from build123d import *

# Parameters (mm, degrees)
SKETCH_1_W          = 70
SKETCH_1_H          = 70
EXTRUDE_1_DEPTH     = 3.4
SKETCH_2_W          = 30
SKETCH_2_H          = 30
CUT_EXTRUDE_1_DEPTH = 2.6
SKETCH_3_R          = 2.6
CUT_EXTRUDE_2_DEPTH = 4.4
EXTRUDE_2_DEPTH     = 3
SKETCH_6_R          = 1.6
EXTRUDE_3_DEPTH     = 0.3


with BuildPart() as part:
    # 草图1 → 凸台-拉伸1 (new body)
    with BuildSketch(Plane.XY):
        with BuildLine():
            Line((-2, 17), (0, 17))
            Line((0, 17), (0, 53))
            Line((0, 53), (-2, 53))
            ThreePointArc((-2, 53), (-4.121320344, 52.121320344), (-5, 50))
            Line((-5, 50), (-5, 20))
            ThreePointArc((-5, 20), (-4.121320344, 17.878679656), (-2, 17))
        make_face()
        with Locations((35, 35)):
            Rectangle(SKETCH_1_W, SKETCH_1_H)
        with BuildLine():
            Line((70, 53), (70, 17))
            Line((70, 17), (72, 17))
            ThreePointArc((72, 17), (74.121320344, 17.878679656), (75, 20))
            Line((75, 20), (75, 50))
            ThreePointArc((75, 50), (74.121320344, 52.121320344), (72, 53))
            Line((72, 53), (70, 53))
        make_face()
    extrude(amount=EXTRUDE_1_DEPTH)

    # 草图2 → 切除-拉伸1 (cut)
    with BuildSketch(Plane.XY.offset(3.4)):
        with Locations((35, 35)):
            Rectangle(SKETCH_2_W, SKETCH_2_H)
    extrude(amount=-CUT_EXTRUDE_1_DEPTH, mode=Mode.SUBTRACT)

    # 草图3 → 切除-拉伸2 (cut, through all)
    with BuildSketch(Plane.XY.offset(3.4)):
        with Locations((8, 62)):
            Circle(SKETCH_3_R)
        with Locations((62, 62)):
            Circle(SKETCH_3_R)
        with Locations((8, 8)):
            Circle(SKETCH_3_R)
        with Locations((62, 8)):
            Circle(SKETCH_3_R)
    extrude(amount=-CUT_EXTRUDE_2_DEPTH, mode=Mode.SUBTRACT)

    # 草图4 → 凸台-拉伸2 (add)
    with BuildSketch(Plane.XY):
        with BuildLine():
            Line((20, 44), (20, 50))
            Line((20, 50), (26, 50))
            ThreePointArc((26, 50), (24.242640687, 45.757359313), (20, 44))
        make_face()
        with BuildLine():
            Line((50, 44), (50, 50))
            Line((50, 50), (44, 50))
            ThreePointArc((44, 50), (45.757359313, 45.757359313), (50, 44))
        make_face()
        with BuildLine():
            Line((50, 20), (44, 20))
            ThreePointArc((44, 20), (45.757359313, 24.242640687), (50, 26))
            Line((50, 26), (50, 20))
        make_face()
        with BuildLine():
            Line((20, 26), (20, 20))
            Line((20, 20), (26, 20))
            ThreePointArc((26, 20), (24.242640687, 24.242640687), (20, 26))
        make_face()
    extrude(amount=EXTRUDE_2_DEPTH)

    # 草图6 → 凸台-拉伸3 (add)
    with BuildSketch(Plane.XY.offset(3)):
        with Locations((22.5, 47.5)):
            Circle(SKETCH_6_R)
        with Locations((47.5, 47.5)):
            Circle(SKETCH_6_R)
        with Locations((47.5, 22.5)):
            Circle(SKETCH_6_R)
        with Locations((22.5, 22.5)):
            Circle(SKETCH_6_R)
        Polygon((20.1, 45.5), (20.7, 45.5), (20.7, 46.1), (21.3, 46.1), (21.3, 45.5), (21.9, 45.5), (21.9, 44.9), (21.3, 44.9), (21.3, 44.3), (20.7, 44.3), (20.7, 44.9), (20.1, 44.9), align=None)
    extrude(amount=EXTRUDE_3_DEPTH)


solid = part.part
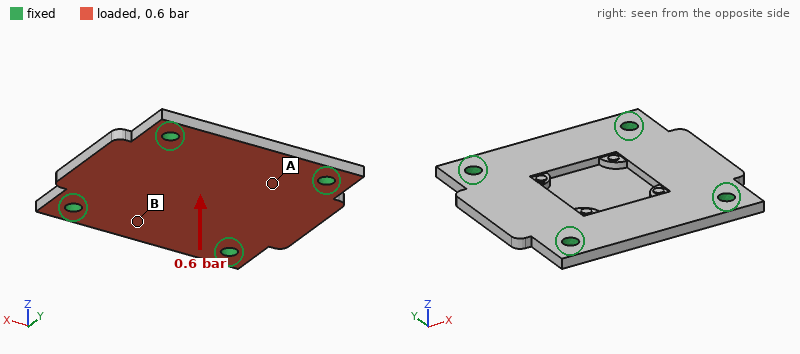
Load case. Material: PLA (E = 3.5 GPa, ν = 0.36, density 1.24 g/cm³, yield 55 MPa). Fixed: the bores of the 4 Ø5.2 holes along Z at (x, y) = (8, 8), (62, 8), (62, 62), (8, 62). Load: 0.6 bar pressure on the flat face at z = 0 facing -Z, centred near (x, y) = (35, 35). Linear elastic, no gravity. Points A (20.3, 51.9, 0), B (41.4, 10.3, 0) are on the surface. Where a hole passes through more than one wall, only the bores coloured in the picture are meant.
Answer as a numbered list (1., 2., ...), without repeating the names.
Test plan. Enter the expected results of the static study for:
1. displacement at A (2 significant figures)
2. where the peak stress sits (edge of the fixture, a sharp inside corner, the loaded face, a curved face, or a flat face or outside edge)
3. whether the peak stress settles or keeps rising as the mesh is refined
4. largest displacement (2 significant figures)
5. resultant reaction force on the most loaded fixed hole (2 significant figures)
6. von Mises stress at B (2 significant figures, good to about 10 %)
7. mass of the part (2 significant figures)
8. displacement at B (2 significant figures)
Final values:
1. 0.15 mm
2. edge of the fixture
3. keeps rising
4. 0.66 mm
5. 84 N
6. 3.6 MPa
7. 19 g
8. 0.14 mm
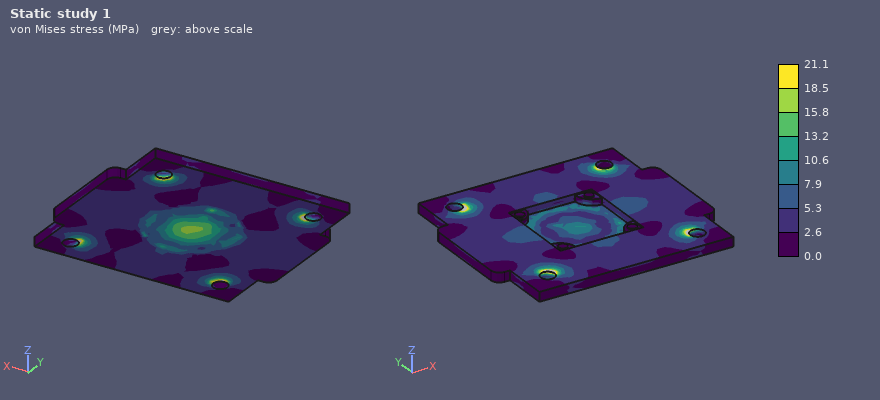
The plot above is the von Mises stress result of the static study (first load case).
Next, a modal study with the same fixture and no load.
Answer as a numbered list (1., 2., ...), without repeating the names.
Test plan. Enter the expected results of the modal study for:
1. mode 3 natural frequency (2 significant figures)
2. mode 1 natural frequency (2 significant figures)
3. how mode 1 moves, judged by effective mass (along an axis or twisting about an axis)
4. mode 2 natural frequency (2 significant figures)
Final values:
1. 2000 Hz
2. 1700 Hz
3. along Z
4. 2000 Hz
